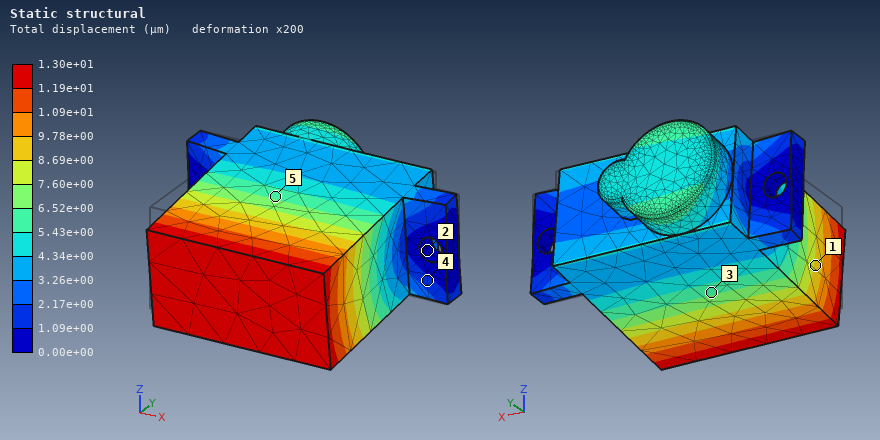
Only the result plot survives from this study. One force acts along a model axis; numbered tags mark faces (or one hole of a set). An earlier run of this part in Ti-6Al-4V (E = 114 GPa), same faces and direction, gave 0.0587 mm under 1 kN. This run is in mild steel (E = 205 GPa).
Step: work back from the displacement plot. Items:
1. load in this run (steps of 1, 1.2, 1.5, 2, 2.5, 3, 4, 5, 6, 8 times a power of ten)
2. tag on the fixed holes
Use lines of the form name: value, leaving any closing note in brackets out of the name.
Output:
load in this run: 400 N
tag on the fixed holes: 2
